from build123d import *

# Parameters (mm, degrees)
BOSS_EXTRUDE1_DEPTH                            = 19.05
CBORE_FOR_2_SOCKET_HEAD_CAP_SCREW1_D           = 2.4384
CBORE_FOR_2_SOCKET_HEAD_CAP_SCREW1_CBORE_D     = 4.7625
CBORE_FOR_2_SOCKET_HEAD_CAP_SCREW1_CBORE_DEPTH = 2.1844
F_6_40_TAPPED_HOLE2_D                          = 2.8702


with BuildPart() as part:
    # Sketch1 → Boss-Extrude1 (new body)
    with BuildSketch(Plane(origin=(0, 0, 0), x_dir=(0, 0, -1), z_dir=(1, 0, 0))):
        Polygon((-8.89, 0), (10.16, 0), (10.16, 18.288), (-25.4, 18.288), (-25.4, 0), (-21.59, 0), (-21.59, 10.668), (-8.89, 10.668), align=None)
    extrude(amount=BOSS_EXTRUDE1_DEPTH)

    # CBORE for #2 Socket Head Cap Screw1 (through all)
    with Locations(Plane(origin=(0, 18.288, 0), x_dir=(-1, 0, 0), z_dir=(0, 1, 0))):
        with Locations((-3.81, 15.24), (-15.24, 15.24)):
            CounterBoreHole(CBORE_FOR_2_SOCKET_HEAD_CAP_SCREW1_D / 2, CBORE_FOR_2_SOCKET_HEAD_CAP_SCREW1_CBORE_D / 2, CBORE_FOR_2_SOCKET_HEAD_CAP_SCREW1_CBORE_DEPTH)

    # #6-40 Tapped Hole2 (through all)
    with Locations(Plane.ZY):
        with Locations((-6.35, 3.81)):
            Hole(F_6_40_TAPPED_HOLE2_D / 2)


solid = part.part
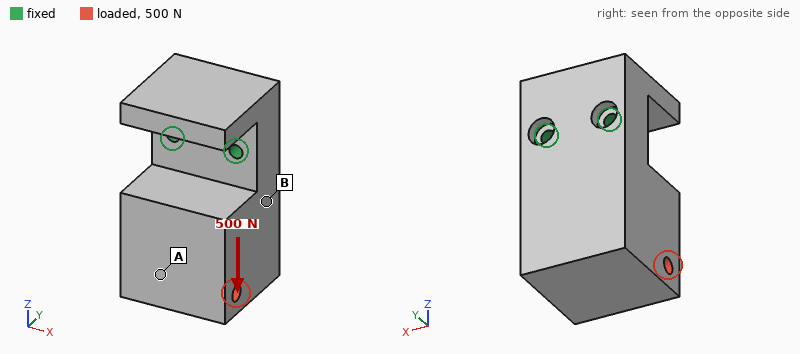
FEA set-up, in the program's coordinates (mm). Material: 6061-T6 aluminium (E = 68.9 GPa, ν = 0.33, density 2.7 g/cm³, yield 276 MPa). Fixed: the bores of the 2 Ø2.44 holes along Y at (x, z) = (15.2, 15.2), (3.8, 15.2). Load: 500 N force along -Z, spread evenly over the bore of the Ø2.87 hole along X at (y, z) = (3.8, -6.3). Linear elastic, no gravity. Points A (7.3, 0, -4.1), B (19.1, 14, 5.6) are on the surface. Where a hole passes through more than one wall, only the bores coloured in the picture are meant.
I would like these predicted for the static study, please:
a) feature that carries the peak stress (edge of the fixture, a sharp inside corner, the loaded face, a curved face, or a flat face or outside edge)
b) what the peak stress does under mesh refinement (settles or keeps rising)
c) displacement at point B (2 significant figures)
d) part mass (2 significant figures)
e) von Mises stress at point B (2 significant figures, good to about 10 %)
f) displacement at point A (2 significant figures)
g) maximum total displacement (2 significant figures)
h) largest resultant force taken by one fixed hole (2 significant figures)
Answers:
edge of the fixture
keeps rising
8.6 µm
26 g
11 MPa
32 µm
39 µm
260 N
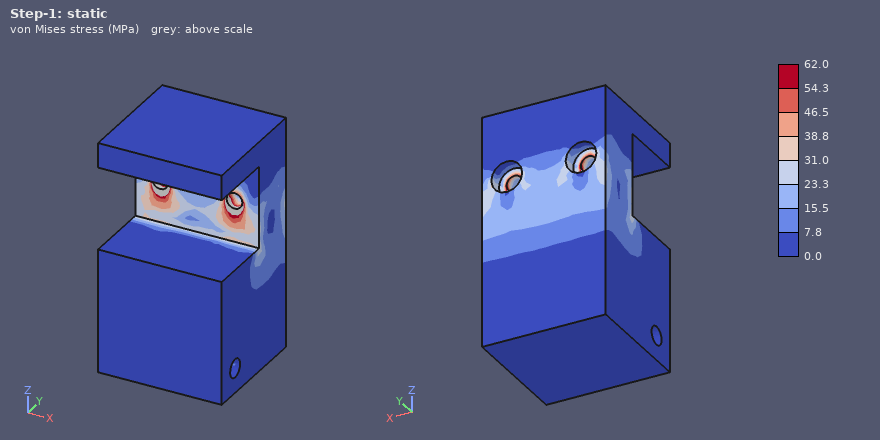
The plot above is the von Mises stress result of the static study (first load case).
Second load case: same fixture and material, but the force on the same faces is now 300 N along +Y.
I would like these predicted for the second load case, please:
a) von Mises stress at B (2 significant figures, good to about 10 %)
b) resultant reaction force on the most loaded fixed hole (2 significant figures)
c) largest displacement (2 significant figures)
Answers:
11 MPa
160 N
44 µm
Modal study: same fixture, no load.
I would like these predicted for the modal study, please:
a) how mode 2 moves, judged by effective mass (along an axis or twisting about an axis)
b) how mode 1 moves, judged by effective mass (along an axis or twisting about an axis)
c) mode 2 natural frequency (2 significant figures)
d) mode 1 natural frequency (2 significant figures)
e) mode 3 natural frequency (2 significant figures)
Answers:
along X
along Y
9500 Hz
4400 Hz
15 kHz
